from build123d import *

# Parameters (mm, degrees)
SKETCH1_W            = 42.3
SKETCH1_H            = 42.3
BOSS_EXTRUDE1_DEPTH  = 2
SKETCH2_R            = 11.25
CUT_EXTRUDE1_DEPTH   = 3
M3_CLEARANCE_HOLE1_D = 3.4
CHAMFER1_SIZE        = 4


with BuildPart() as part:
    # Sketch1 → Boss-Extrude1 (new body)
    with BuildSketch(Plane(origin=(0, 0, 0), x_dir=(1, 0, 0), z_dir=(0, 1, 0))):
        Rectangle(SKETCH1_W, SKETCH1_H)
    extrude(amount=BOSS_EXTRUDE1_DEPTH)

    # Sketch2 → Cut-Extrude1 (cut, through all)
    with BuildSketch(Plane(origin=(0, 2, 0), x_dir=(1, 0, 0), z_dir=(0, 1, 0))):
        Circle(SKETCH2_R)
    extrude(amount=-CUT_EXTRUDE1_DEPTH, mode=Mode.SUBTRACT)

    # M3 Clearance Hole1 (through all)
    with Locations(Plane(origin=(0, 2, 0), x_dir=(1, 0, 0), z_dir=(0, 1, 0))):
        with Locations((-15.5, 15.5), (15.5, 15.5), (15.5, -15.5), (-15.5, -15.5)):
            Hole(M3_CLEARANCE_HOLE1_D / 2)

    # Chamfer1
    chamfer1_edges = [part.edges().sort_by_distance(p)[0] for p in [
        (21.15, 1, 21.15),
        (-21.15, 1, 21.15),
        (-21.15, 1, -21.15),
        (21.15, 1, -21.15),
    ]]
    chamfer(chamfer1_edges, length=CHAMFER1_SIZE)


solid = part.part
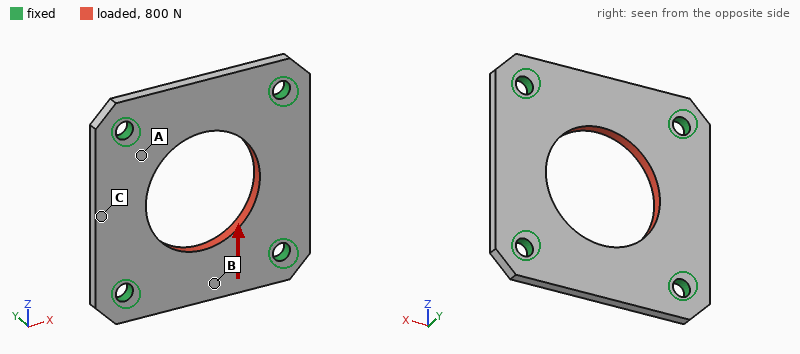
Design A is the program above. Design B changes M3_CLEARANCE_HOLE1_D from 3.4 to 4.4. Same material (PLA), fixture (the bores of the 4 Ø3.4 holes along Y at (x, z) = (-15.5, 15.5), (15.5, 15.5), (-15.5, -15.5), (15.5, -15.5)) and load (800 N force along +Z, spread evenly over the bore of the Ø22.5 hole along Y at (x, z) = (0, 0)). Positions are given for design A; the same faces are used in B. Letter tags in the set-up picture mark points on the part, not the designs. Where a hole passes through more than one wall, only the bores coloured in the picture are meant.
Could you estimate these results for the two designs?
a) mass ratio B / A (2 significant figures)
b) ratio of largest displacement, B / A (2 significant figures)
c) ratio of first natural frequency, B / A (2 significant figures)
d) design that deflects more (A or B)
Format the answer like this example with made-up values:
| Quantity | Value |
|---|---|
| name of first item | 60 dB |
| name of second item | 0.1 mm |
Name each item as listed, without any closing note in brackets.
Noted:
| Quantity | Value |
|---|---|
| mass ratio B / A | 0.98 |
| ratio of largest displacement, B / A | 0.92 |
| ratio of first natural frequency, B / A | 1.1 |
| design that deflects more | A |
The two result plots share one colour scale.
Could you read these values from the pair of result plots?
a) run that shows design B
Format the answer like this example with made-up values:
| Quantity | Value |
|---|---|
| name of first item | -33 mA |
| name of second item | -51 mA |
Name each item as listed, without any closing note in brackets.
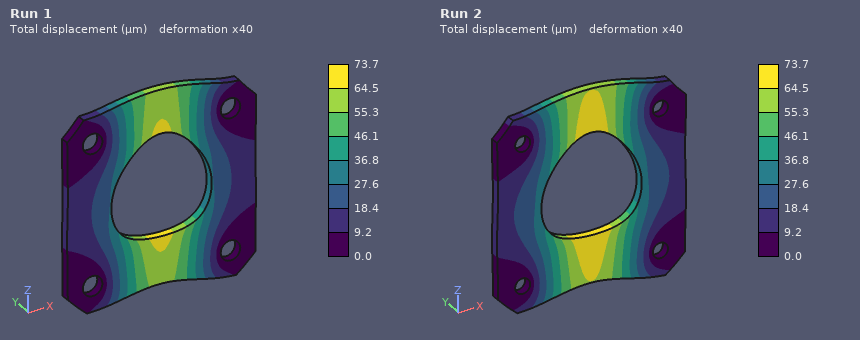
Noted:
| Quantity | Value |
|---|---|
| run that shows design B | Run 1 |
